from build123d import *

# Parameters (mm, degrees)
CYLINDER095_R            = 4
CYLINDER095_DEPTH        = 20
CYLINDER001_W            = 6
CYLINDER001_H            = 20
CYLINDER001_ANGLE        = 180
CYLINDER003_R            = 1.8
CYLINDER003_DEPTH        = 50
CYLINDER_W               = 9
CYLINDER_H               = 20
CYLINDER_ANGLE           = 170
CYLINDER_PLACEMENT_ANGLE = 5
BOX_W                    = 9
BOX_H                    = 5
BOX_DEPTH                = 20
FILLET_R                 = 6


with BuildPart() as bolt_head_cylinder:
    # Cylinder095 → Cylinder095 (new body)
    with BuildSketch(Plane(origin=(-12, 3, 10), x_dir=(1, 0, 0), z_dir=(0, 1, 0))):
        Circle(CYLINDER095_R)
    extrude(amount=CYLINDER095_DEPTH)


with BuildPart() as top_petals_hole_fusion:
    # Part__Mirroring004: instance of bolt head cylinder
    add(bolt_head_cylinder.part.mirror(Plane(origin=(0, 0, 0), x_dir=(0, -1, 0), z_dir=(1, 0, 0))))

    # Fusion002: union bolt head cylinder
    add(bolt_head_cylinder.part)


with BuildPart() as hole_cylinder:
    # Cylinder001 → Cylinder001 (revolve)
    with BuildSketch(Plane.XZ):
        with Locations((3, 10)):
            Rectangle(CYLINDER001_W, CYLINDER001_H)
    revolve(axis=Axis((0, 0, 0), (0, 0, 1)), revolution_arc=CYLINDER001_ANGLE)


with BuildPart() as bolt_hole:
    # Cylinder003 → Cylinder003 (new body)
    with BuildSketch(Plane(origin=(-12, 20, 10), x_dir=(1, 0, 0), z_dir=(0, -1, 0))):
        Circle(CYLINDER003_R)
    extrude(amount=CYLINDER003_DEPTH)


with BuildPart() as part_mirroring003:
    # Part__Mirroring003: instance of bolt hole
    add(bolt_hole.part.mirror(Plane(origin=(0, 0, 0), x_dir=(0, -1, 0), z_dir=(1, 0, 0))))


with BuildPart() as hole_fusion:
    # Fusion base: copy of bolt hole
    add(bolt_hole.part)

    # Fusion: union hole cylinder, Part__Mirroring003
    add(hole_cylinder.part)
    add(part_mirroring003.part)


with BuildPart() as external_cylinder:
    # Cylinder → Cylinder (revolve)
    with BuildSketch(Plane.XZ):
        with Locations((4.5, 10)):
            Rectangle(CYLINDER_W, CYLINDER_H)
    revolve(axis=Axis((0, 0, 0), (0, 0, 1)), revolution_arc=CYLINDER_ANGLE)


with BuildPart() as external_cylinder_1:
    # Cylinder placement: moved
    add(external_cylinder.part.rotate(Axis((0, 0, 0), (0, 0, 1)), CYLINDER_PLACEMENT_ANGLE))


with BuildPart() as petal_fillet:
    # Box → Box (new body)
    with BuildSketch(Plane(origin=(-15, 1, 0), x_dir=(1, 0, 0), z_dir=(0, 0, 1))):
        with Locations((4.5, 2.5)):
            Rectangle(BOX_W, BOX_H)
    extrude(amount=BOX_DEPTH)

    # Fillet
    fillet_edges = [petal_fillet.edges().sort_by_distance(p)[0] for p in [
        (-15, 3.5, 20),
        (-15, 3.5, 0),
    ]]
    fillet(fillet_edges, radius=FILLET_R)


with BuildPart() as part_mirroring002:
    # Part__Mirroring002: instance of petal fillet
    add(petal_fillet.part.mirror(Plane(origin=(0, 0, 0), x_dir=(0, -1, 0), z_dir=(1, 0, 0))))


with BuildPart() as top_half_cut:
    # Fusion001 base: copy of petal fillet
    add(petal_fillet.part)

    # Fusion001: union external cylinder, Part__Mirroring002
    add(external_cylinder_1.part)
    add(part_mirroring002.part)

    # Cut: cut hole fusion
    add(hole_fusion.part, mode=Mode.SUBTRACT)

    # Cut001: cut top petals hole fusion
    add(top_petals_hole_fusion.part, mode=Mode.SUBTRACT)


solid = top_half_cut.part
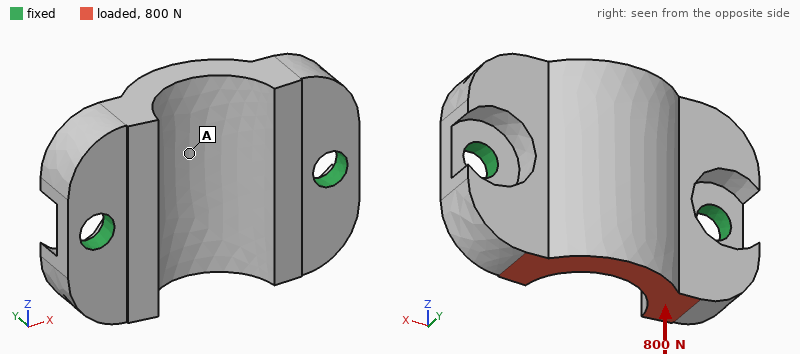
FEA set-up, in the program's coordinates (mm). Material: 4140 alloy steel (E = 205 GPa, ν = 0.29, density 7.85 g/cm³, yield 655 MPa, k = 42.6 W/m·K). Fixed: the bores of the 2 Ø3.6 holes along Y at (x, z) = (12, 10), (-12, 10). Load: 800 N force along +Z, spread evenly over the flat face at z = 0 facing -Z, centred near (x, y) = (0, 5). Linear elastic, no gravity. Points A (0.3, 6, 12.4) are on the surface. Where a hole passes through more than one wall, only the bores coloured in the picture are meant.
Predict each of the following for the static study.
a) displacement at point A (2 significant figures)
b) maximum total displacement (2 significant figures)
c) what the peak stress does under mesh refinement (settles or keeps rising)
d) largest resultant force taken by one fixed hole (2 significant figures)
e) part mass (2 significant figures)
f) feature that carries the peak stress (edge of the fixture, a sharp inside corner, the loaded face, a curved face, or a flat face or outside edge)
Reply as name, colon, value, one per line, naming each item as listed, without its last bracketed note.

displacement at point A: 5.7 µm
maximum total displacement: 14 µm
what the peak stress does under mesh refinement: keeps rising
largest resultant force taken by one fixed hole: 400 N
part mass: 18 g
feature that carries the peak stress: edge of the fixture
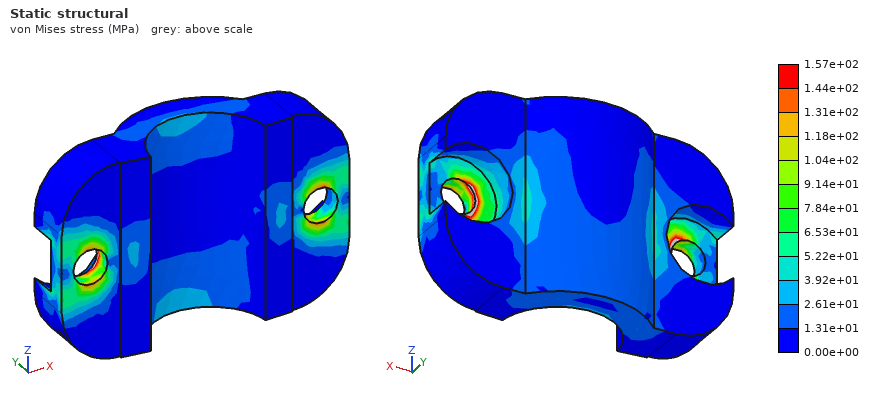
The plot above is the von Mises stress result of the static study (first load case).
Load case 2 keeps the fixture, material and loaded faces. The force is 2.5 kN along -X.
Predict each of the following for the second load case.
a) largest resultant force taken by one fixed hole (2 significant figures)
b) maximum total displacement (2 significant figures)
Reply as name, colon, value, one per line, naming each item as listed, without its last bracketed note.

largest resultant force taken by one fixed hole: 1.5 kN
maximum total displacement: 15 µm
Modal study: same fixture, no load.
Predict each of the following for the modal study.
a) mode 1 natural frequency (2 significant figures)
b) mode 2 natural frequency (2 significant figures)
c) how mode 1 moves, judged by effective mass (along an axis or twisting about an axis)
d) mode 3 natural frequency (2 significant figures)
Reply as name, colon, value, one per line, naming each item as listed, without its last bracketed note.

mode 1 natural frequency: 10 kHz
mode 2 natural frequency: 25 kHz
how mode 1 moves, judged by effective mass: along Z
mode 3 natural frequency: 25 kHz
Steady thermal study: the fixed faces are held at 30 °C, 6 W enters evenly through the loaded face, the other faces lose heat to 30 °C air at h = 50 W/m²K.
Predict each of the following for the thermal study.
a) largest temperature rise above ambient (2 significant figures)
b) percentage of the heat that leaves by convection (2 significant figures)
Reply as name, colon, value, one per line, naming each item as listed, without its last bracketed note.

largest temperature rise above ambient: 23 K
percentage of the heat that leaves by convection: 11 %
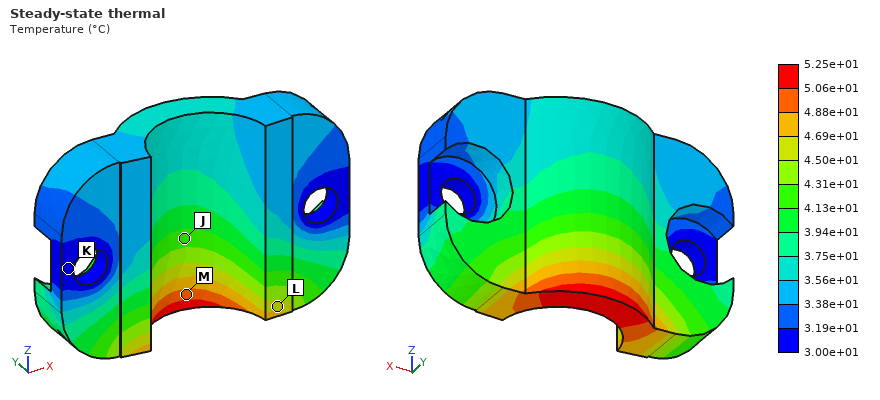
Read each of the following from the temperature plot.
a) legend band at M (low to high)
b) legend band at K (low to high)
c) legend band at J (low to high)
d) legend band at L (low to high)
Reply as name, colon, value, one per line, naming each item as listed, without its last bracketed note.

legend band at M: 4.88e+01 to 5.06e+01 °C
legend band at K: 3.00e+01 to 3.19e+01 °C
legend band at J: 4.13e+01 to 4.31e+01 °C
legend band at L: 4.50e+01 to 4.69e+01 °C
